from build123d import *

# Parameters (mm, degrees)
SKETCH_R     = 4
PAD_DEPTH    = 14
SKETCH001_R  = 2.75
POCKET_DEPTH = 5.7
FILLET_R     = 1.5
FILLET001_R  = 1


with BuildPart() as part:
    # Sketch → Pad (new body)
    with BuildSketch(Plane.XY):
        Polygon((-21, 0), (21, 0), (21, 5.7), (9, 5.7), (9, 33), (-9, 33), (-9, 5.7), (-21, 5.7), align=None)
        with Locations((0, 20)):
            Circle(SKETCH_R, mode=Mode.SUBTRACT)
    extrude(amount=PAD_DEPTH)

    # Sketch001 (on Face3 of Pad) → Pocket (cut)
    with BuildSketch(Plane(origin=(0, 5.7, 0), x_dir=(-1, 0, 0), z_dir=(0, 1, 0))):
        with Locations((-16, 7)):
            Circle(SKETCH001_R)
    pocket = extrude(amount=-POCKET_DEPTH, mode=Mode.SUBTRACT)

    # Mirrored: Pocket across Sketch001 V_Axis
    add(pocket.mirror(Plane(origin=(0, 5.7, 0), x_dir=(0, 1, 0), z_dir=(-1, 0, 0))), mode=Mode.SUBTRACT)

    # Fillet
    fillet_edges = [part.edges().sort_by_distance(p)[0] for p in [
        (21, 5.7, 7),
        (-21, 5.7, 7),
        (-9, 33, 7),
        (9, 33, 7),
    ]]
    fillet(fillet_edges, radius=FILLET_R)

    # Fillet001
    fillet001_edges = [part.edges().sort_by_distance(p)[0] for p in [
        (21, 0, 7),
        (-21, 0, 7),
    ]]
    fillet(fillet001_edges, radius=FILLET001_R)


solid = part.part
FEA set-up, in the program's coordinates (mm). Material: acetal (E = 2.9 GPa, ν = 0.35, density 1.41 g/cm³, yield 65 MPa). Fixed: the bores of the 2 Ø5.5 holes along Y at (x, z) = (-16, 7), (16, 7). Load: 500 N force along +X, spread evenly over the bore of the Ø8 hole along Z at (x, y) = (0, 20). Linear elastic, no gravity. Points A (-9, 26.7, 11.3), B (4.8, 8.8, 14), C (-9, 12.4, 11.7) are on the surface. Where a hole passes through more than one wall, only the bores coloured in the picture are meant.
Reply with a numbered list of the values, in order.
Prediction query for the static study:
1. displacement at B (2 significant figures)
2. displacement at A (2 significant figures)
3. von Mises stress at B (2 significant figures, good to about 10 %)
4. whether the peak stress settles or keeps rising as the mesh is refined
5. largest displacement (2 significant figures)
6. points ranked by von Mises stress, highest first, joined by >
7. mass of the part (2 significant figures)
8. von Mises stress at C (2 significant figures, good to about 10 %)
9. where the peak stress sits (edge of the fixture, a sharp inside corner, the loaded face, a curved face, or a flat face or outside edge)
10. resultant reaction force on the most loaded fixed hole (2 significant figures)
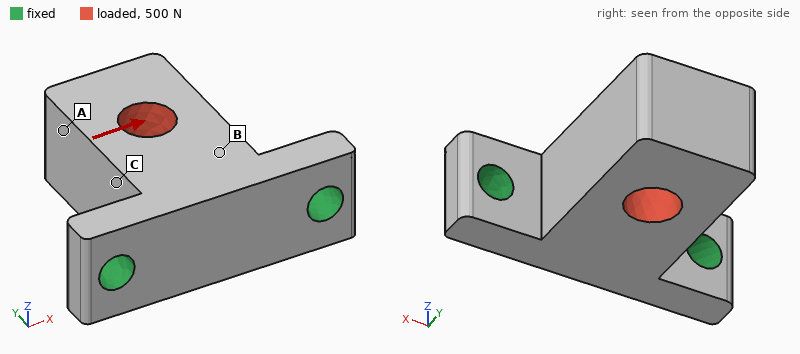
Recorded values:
1. 0.047 mm
2. 0.23 mm
3. 4.4 MPa
4. keeps rising
5. 0.28 mm
6. C > B > A
7. 13 g
8. 6.2 MPa
9. edge of the fixture
10. 440 N
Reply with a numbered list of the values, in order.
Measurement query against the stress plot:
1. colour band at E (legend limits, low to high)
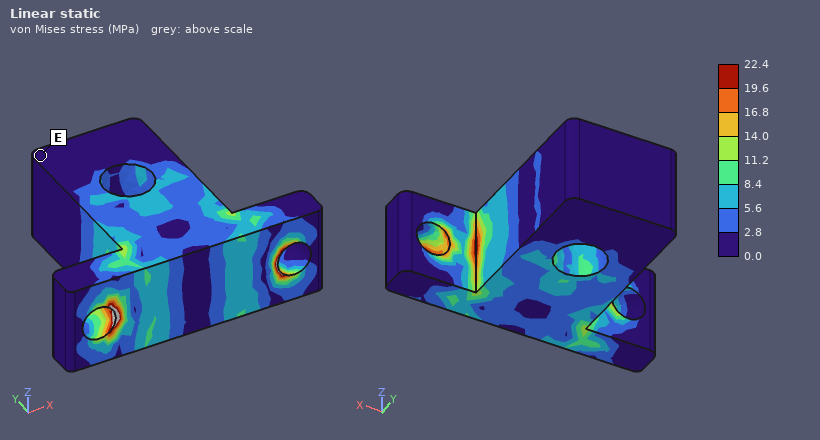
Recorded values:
1. 0.0 to 2.8 MPa
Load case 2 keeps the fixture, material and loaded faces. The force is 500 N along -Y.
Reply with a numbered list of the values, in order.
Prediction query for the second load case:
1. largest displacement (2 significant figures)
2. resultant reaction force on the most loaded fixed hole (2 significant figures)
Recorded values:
1. 61 µm
2. 270 N
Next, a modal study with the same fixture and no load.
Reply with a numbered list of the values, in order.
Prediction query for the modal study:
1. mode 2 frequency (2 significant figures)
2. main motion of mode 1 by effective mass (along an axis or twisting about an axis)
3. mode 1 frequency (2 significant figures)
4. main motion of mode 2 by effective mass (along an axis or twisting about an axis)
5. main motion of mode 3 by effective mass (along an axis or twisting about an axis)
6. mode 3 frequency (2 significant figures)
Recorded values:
1. 2700 Hz
2. along Z
3. 1300 Hz
4. along X
5. along Y
6. 4800 Hz
